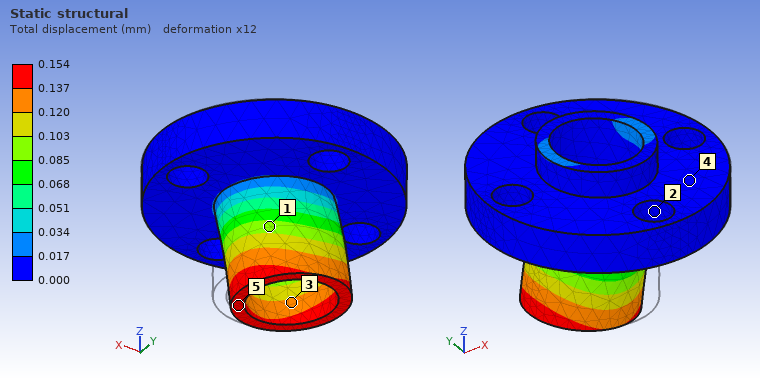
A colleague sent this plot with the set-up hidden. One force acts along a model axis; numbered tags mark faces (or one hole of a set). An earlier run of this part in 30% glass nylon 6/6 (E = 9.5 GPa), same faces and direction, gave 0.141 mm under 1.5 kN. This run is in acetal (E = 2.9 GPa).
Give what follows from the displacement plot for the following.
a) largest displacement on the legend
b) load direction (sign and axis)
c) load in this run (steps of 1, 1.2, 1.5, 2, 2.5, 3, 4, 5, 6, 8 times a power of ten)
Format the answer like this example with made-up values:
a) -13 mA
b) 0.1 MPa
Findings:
a) 0.154 mm
b) -X
c) 500 N
